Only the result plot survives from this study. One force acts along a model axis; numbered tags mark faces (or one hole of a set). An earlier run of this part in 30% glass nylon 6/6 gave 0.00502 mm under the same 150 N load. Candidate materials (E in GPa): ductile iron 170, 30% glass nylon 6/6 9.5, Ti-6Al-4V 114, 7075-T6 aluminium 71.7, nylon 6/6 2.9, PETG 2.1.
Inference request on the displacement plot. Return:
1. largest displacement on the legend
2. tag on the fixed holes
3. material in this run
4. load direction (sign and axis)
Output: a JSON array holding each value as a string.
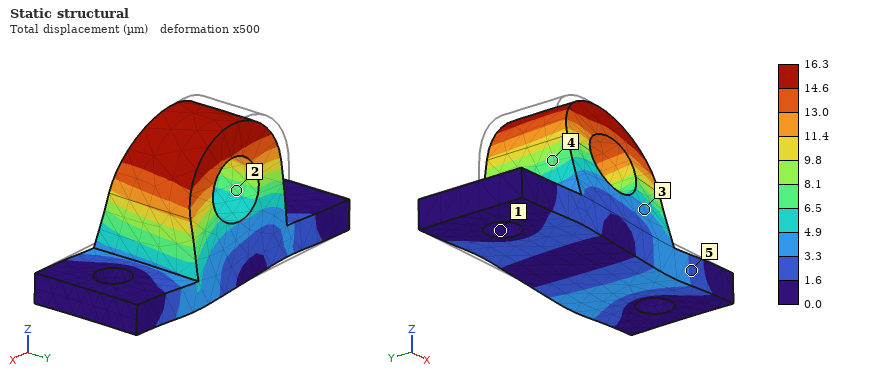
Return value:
["16.3 µm", "1", "nylon 6/6", "+X"]
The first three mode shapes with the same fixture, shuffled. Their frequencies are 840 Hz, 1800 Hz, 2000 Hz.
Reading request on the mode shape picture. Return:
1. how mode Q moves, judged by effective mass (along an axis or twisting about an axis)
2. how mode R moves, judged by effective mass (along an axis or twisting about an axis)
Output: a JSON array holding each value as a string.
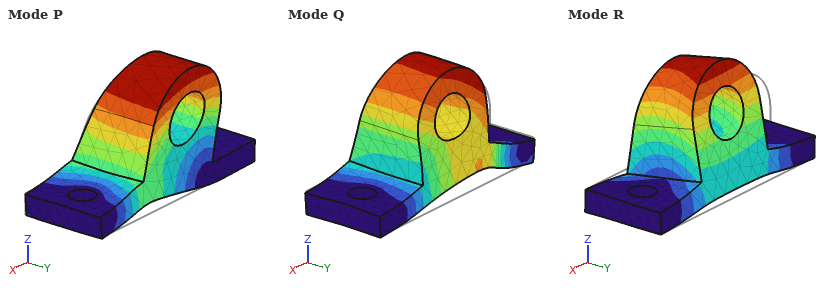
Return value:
["along Z", "along Y"]
